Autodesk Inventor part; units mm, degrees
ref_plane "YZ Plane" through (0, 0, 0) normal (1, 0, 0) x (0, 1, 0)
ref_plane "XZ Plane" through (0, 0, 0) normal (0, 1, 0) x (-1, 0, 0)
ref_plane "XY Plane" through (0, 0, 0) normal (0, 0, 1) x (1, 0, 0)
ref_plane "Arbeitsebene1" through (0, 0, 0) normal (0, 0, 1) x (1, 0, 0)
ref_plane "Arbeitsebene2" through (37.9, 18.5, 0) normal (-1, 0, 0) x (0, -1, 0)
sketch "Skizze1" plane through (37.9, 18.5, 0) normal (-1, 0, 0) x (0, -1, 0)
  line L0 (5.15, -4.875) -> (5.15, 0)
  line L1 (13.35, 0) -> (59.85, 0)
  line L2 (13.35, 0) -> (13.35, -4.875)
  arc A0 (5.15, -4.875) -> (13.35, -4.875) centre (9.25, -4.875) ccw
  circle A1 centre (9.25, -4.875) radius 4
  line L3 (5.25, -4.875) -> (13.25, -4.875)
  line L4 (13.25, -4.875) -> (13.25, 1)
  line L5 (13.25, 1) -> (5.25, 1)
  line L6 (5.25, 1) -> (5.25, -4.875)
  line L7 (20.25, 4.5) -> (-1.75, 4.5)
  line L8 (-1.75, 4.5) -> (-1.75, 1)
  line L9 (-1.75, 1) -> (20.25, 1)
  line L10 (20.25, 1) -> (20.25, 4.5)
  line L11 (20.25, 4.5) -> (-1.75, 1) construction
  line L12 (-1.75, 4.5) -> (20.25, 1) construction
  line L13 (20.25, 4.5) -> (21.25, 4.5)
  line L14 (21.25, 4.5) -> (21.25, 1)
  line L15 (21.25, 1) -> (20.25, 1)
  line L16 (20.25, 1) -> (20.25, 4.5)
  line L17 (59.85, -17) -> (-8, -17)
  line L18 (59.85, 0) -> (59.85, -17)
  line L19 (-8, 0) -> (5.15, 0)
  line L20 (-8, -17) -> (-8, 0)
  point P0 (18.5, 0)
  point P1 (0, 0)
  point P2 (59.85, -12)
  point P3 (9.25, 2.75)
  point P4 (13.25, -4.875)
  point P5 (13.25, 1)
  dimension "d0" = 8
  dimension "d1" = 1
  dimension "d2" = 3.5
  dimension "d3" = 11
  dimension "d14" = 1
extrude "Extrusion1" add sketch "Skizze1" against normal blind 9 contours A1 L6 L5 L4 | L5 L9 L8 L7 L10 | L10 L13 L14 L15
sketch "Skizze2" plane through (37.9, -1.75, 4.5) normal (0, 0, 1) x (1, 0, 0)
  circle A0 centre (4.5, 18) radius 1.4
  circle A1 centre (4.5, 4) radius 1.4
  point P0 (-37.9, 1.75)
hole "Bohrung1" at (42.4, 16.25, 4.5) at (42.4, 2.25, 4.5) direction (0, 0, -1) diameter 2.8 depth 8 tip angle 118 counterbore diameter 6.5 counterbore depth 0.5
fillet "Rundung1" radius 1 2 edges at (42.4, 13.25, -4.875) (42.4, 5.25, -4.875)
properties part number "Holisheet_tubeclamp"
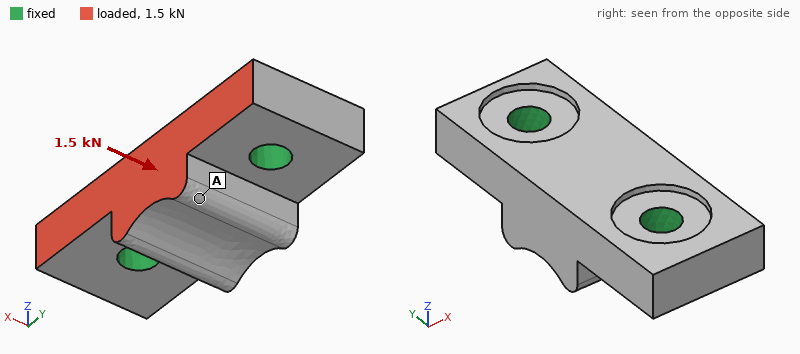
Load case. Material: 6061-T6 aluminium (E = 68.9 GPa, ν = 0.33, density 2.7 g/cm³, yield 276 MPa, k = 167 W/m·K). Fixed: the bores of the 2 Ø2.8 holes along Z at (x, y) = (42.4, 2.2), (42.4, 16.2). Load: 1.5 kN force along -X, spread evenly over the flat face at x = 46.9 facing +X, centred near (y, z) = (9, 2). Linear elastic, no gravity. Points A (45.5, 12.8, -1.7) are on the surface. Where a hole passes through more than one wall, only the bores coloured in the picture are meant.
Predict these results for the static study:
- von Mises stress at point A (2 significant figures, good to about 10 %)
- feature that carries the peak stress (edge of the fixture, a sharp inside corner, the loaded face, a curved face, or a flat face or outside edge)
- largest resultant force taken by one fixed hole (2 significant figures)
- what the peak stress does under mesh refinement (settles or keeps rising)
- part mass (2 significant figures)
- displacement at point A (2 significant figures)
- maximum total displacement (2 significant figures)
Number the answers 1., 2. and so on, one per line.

1. 15 MPa
2. edge of the fixture
3. 790 N
4. keeps rising
5. 2.2 g
6. 5.5 µm
7. 6.2 µm
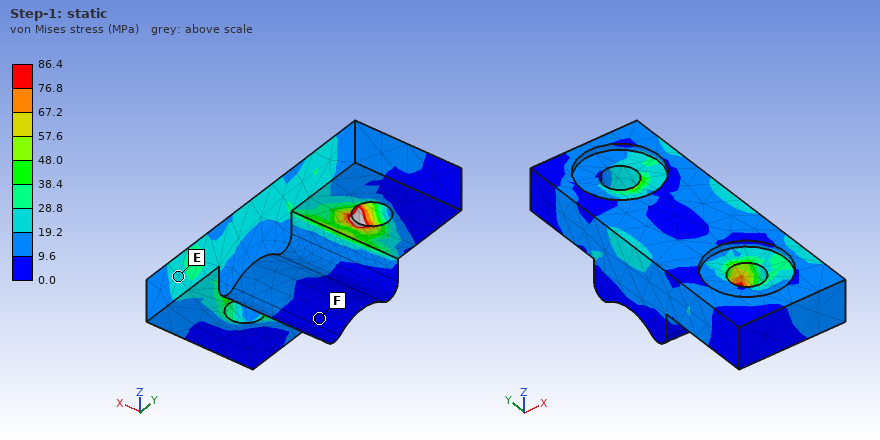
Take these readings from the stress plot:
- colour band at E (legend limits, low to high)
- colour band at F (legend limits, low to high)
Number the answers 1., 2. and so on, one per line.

1. 19.2 to 28.8 MPa
2. 0.0 to 9.6 MPa
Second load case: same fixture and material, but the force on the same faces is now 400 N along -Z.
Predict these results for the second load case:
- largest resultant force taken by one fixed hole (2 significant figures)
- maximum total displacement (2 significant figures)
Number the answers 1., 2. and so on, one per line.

1. 210 N
2. 6.8 µm
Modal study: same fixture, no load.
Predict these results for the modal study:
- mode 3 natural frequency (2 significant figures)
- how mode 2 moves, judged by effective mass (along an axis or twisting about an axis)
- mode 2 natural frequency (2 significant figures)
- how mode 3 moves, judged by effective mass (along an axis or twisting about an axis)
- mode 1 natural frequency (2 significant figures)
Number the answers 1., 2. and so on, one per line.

1. 77 kHz
2. along Z
3. 63 kHz
4. along X
5. 50 kHz
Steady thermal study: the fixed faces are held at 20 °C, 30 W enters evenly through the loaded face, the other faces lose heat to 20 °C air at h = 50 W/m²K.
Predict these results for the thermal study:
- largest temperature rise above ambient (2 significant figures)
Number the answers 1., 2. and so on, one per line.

1. 14 K
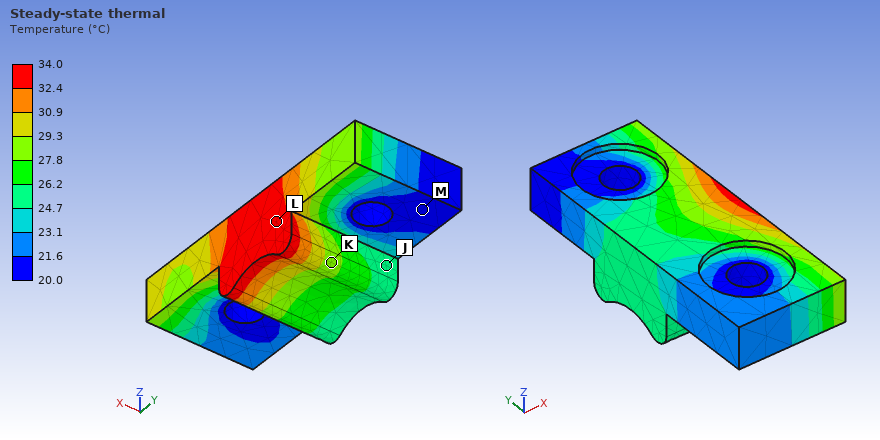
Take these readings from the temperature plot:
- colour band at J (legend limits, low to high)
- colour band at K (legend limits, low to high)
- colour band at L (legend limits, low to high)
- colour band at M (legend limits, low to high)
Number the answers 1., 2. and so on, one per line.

1. 24.7 to 26.2 °C
2. 27.8 to 29.3 °C
3. 32.4 to 34.0 °C
4. 20.0 to 21.6 °C
